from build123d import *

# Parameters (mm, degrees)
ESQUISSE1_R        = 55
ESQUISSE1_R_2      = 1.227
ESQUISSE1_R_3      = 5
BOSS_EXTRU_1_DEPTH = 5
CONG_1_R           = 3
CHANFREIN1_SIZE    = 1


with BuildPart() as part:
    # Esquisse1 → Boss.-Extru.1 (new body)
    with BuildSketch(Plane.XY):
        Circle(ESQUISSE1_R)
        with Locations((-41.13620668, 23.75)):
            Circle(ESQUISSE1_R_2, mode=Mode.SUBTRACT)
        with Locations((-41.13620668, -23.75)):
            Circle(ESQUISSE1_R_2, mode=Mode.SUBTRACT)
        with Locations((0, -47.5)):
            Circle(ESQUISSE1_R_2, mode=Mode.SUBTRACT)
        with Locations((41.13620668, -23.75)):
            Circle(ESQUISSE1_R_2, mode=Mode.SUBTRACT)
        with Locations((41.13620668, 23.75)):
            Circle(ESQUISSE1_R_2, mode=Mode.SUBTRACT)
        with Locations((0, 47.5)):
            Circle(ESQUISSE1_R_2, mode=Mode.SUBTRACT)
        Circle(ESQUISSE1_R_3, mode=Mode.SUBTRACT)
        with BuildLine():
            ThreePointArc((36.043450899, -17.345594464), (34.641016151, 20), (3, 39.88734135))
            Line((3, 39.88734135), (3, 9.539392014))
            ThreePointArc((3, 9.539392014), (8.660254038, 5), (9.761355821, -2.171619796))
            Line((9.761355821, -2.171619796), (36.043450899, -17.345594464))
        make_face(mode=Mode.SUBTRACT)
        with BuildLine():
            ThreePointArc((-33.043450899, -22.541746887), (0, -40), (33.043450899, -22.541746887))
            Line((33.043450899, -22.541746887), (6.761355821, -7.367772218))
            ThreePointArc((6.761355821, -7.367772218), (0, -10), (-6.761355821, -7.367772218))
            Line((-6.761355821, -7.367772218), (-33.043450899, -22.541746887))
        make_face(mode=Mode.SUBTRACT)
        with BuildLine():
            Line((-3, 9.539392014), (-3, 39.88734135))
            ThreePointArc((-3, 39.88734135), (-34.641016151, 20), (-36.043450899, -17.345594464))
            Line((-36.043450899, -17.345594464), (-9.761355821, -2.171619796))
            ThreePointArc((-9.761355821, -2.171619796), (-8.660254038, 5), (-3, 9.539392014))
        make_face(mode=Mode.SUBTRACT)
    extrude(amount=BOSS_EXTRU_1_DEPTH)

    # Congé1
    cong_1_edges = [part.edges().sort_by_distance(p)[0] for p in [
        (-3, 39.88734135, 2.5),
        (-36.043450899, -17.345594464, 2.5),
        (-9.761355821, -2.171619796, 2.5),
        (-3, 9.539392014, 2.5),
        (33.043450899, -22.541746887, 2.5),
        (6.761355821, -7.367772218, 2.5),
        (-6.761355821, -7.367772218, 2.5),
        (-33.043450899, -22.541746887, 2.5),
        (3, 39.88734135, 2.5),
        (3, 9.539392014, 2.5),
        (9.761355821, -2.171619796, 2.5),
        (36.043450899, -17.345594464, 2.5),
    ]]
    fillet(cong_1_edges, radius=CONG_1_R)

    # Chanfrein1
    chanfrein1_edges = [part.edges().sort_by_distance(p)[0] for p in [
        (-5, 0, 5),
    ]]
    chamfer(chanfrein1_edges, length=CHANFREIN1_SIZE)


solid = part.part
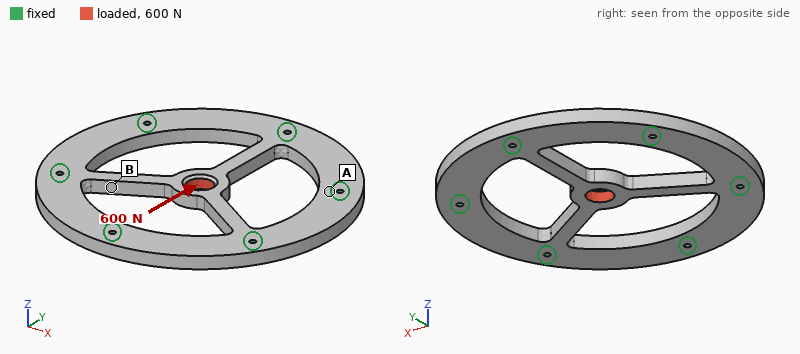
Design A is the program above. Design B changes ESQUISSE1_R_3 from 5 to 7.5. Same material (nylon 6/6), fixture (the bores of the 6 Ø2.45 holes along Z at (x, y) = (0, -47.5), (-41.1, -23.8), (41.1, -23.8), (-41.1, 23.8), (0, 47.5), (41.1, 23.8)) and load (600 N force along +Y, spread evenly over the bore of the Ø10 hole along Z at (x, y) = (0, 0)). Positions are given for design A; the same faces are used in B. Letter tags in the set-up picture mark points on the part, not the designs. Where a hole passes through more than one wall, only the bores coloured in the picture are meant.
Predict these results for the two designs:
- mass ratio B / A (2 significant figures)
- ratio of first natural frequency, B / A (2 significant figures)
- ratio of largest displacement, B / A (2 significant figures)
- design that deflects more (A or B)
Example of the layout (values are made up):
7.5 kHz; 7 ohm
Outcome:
0.98; 1.0; 3.3; B
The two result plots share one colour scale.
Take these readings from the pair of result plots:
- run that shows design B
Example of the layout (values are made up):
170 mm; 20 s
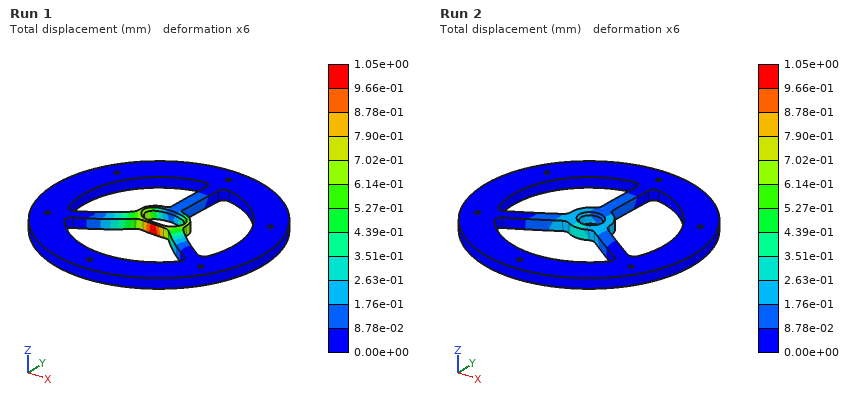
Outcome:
Run 1
